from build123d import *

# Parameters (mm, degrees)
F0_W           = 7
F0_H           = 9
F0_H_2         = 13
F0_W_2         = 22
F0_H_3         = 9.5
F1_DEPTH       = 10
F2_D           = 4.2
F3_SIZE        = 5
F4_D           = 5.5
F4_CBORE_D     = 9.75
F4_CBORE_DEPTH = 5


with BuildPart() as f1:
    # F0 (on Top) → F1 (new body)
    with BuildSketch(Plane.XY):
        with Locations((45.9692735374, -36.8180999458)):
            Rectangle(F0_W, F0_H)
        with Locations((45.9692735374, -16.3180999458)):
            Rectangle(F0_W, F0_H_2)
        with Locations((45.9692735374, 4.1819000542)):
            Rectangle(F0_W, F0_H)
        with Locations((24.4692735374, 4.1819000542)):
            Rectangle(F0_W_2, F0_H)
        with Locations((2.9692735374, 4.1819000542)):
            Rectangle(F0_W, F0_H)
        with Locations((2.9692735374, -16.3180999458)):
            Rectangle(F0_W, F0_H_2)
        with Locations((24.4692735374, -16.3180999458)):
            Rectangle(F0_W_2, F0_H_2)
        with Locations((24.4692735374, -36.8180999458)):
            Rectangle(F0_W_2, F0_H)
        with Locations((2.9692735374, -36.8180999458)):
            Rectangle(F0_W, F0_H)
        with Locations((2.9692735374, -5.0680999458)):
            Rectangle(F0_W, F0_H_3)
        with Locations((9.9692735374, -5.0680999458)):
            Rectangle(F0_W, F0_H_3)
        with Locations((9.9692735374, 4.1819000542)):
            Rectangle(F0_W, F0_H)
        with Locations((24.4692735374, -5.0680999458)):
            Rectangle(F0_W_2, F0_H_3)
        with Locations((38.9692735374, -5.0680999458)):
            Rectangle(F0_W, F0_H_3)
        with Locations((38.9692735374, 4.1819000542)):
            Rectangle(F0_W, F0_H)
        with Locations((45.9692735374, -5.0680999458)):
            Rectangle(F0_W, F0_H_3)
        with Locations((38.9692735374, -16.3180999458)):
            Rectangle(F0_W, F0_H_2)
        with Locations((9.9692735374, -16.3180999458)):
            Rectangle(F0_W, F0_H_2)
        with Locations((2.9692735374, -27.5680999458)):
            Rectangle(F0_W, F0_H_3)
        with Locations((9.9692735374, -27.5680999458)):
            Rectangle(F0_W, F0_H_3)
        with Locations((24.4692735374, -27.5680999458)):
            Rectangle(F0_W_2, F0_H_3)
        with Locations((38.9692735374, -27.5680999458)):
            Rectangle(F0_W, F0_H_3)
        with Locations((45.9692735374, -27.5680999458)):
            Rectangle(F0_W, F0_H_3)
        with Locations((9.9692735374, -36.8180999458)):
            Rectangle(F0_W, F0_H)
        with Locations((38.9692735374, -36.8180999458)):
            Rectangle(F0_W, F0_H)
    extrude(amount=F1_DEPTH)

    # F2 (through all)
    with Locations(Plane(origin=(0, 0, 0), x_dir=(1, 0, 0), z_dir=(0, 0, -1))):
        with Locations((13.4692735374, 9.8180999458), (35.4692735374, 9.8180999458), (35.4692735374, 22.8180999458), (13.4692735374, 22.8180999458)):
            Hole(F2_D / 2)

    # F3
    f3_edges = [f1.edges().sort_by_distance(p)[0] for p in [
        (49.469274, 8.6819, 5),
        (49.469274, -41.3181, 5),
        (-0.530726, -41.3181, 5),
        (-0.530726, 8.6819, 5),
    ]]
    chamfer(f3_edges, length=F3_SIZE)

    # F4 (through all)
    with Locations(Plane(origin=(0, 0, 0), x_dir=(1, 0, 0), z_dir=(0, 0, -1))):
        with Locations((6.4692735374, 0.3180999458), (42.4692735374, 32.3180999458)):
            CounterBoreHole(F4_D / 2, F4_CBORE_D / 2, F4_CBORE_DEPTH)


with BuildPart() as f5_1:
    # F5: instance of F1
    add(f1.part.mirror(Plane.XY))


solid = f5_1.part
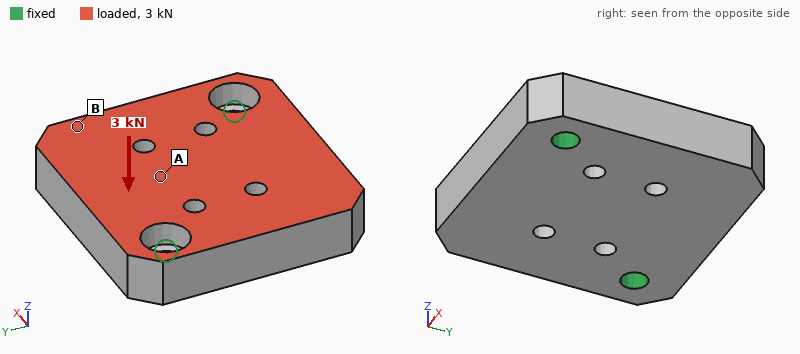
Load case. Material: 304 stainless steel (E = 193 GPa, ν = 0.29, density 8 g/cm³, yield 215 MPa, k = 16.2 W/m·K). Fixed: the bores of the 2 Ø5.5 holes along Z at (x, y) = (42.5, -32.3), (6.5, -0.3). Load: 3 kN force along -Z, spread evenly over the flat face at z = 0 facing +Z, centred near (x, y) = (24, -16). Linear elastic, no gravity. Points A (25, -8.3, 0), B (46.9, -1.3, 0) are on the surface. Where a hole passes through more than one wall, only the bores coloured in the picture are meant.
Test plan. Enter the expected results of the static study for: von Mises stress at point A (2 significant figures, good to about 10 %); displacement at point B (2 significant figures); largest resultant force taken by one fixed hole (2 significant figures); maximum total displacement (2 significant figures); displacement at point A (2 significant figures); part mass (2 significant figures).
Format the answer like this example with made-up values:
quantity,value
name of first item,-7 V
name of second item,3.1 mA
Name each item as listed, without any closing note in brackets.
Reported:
quantity,value
von Mises stress at point A,25 MPa
displacement at point B,10 µm
largest resultant force taken by one fixed hole,1.8 kN
maximum total displacement,12 µm
displacement at point A,5.4 µm
part mass,180 g
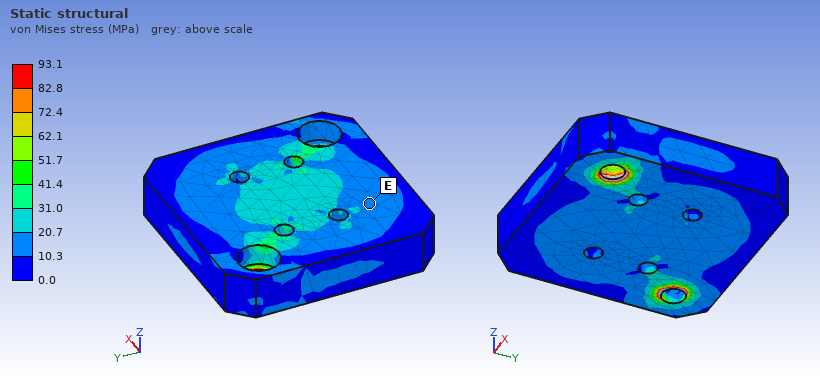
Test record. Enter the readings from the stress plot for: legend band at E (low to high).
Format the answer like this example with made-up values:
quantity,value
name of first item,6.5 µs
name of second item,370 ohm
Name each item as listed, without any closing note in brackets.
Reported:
quantity,value
legend band at E,10.3 to 20.7 MPa
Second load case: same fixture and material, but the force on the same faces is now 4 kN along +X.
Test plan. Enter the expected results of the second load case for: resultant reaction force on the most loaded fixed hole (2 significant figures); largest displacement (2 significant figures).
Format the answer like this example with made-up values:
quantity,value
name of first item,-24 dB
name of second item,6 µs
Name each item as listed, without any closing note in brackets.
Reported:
quantity,value
resultant reaction force on the most loaded fixed hole,2.0 kN
largest displacement,21 µm
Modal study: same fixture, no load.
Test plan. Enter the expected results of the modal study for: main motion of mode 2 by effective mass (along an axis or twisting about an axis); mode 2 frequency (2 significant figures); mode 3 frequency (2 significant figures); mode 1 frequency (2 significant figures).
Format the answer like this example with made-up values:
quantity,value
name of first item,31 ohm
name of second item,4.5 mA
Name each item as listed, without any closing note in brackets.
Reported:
quantity,value
main motion of mode 2 by effective mass,along Z
mode 2 frequency,7700 Hz
mode 3 frequency,19 kHz
mode 1 frequency,4500 Hz
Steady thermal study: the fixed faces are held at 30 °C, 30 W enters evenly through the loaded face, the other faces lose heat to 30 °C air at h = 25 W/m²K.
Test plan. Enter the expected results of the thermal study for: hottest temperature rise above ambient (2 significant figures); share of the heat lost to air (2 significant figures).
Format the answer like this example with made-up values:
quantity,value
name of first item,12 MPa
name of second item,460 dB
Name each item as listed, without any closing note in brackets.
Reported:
quantity,value
hottest temperature rise above ambient,63 K
share of the heat lost to air,18 %
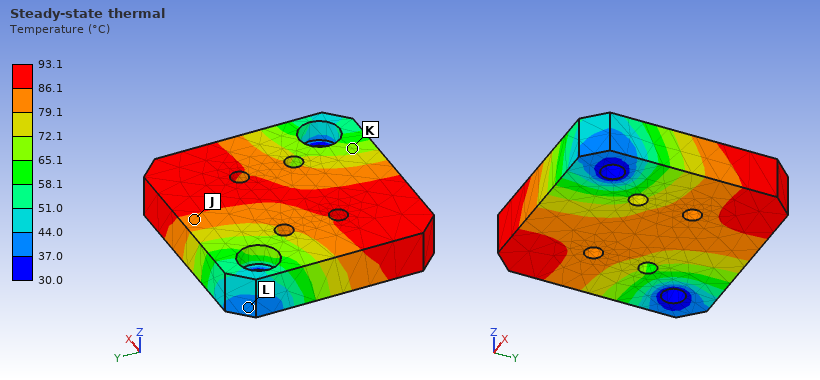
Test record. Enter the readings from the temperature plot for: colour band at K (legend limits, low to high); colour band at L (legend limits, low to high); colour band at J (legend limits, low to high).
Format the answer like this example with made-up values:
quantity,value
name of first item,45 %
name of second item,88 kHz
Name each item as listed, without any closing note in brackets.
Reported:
quantity,value
colour band at K,65.1 to 72.1 °C
colour band at L,37.0 to 44.0 °C
colour band at J,79.1 to 86.1 °C
